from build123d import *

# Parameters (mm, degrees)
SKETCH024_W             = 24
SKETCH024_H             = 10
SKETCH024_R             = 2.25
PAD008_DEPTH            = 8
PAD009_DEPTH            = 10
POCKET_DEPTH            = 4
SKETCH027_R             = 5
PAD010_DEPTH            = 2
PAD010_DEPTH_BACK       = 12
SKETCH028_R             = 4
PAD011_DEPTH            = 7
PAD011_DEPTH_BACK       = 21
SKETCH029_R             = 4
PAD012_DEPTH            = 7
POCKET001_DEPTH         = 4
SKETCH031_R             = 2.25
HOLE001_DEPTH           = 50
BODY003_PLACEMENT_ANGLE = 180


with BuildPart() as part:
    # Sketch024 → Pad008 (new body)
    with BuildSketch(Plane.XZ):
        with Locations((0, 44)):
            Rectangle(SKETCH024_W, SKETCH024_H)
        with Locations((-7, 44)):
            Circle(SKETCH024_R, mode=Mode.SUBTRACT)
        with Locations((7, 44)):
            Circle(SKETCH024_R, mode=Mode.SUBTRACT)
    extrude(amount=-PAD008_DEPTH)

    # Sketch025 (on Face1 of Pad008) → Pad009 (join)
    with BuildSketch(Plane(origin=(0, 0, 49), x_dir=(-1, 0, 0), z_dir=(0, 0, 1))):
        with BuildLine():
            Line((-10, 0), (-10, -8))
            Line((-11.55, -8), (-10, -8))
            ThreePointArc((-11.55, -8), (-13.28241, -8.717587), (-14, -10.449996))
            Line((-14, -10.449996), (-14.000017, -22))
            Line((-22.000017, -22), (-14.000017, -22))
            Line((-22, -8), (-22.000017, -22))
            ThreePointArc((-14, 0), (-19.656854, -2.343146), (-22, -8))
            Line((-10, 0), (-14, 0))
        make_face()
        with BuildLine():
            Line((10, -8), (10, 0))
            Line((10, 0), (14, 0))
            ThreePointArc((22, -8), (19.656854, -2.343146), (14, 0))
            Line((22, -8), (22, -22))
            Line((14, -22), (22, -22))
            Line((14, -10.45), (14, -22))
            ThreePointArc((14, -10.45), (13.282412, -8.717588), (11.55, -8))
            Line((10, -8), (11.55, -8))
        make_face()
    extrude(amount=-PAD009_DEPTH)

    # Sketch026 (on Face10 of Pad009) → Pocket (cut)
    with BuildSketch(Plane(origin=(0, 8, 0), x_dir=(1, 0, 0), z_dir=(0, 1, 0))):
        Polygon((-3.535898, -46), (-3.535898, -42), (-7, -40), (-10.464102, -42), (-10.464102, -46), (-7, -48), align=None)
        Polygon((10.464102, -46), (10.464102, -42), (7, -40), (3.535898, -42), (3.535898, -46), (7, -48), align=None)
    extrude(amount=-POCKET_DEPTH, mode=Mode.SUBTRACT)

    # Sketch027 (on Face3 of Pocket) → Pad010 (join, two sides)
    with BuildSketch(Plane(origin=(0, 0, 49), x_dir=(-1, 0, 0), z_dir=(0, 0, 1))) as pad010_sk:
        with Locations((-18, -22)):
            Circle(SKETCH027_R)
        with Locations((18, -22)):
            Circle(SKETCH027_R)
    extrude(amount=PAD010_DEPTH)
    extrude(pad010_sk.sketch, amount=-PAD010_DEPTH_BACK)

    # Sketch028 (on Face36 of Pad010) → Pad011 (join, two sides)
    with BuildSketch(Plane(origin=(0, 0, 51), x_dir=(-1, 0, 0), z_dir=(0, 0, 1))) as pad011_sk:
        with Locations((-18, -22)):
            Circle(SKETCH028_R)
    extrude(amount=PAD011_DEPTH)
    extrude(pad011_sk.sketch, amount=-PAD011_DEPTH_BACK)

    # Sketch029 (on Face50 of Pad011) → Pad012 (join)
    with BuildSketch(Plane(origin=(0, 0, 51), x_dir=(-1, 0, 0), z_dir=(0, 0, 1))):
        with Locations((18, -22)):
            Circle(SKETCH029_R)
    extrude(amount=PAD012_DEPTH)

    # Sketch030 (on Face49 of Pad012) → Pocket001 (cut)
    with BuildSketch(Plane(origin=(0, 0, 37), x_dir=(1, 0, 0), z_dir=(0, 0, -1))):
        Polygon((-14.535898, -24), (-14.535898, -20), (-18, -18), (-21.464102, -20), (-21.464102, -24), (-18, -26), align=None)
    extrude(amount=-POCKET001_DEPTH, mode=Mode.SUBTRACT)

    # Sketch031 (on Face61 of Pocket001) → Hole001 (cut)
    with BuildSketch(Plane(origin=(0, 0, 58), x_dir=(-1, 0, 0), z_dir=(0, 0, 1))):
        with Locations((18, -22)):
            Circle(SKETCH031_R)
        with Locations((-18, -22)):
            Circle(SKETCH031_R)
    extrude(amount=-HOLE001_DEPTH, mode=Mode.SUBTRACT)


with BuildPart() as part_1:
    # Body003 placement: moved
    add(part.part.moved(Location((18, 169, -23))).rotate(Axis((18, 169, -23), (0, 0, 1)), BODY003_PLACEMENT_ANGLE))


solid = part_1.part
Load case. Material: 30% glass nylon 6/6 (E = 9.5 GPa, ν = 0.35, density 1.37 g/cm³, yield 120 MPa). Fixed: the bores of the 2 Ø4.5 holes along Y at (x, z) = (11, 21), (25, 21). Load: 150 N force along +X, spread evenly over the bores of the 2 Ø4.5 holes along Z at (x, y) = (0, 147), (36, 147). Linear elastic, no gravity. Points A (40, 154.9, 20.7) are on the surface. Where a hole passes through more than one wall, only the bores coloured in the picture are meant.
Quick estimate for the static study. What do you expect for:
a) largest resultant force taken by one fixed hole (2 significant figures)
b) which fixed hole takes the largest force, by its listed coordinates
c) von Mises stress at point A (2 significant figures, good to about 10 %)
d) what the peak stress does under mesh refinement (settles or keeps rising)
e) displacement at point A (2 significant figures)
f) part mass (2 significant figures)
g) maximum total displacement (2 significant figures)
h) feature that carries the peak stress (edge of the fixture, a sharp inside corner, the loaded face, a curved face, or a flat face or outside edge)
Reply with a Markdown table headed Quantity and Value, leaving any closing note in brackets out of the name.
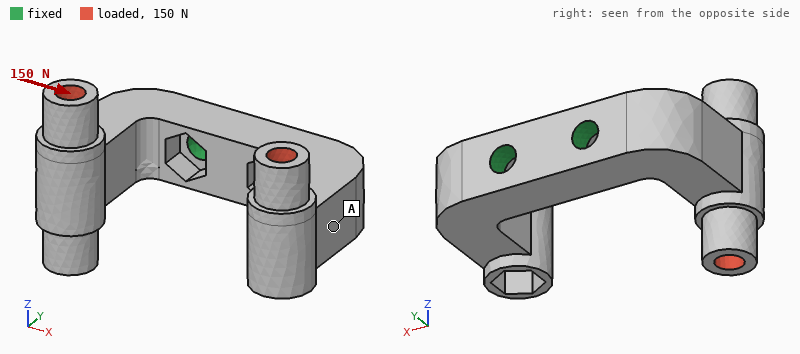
| Quantity | Value |
|---|---|
| largest resultant force taken by one fixed hole | 130 N |
| which fixed hole takes the largest force, by its listed coordinates | (25, 21) |
| von Mises stress at point A | 5.4 MPa |
| what the peak stress does under mesh refinement | keeps rising |
| displacement at point A | 0.078 mm |
| part mass | 9.2 g |
| maximum total displacement | 0.22 mm |
| feature that carries the peak stress | edge of the fixture |
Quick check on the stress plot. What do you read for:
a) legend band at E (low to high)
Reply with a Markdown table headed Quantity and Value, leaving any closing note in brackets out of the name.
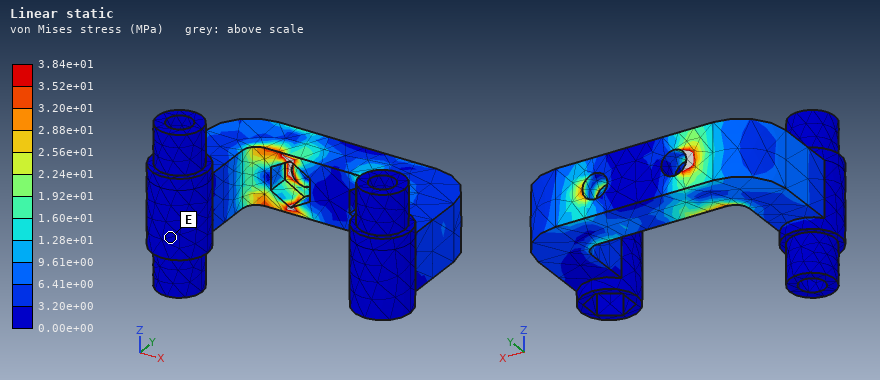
| Quantity | Value |
|---|---|
| legend band at E | 0.00e+00 to 3.20e+00 MPa |
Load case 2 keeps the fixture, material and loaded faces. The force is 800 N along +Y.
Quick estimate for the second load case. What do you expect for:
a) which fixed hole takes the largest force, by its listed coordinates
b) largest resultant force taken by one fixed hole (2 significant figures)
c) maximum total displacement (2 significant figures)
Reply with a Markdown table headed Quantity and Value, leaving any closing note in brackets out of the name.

| Quantity | Value |
|---|---|
| which fixed hole takes the largest force, by its listed coordinates | (11, 21) |
| largest resultant force taken by one fixed hole | 640 N |
| maximum total displacement | 0.41 mm |
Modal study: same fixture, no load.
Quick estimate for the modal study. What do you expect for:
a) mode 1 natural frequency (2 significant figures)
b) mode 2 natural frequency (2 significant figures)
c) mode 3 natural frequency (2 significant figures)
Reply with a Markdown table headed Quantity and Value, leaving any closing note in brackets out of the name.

| Quantity | Value |
|---|---|
| mode 1 natural frequency | 2300 Hz |
| mode 2 natural frequency | 2300 Hz |
| mode 3 natural frequency | 2600 Hz |
